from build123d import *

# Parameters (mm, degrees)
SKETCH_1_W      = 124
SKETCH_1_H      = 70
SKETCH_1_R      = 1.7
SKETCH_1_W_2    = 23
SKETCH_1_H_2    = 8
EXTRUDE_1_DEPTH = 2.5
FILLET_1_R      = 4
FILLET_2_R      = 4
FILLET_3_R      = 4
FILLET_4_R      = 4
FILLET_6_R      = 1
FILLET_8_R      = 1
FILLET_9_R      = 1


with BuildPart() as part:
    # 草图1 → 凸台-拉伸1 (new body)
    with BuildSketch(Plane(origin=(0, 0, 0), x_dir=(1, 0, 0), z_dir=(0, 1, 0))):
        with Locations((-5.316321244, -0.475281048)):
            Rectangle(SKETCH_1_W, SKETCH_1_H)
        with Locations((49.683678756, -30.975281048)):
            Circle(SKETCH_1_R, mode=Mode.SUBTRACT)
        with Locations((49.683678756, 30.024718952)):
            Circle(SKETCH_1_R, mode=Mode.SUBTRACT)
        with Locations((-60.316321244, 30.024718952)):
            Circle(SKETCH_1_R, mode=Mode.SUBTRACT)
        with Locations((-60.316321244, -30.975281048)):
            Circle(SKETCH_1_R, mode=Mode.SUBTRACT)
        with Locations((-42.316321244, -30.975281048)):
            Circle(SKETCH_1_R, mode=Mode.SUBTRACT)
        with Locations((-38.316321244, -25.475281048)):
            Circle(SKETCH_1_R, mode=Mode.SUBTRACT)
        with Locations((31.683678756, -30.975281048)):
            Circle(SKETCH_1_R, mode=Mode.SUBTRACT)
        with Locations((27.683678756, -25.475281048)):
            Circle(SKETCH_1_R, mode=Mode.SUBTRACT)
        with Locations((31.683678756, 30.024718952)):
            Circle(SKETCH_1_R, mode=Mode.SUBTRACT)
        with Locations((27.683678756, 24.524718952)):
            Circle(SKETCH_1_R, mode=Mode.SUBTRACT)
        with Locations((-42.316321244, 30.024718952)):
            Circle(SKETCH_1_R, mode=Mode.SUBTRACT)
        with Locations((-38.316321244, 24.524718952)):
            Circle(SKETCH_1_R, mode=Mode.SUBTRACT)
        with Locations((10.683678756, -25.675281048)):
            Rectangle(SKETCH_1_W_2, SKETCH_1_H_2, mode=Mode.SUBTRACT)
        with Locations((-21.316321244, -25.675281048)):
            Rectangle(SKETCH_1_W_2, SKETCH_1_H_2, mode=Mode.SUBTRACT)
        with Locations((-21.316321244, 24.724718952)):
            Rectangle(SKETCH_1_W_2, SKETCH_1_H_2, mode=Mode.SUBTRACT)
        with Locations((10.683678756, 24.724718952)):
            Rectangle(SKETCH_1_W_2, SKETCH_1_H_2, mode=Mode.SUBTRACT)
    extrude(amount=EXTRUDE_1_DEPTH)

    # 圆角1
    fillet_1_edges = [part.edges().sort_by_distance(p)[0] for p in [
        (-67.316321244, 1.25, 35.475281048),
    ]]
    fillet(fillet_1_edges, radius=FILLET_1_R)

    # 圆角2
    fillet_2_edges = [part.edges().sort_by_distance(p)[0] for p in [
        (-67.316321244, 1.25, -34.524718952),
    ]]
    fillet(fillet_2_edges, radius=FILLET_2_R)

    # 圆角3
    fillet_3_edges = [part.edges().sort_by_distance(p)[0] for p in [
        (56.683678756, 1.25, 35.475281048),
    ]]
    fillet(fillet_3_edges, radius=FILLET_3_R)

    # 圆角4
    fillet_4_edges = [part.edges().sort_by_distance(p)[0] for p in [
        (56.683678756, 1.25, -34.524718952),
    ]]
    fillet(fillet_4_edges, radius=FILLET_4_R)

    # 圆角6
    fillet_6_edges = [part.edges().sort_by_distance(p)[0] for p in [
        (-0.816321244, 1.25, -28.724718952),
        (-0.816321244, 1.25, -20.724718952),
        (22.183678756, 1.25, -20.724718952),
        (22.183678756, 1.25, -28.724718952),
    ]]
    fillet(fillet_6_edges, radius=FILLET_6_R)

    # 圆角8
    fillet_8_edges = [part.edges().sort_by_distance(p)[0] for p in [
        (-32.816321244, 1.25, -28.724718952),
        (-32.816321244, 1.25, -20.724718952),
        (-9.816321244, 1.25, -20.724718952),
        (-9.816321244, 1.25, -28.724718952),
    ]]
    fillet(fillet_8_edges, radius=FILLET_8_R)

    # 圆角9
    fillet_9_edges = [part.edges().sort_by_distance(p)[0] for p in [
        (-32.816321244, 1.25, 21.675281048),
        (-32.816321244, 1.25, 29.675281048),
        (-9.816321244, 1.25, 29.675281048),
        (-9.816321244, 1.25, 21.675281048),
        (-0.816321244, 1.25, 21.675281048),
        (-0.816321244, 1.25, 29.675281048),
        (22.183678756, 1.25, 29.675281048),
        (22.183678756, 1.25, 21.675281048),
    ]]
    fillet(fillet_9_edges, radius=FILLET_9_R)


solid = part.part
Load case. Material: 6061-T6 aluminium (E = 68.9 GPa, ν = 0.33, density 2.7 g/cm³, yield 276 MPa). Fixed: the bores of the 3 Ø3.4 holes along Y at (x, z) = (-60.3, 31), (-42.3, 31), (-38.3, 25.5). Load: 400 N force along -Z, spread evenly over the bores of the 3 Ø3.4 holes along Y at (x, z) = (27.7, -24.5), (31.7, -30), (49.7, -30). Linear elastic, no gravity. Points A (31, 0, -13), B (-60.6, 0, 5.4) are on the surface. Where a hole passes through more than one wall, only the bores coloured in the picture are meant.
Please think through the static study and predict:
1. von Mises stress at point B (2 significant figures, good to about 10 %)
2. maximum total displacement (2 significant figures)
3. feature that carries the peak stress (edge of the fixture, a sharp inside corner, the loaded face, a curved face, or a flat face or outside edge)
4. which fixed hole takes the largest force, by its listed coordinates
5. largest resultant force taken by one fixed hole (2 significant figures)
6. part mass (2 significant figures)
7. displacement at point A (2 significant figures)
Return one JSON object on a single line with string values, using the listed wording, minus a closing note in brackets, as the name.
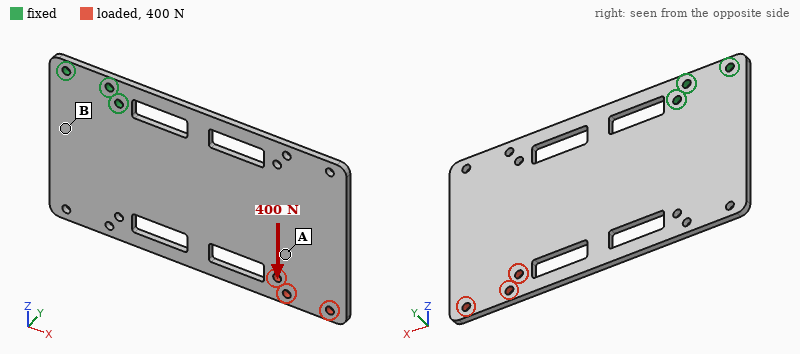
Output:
{"von Mises stress at point B": "20 MPa", "maximum total displacement": "0.18 mm", "feature that carries the peak stress": "a curved face", "which fixed hole takes the largest force, by its listed coordinates": "(-38.3, 25.5)", "largest resultant force taken by one fixed hole": "1.5 kN", "part mass": "53 g", "displacement at point A": "0.13 mm"}
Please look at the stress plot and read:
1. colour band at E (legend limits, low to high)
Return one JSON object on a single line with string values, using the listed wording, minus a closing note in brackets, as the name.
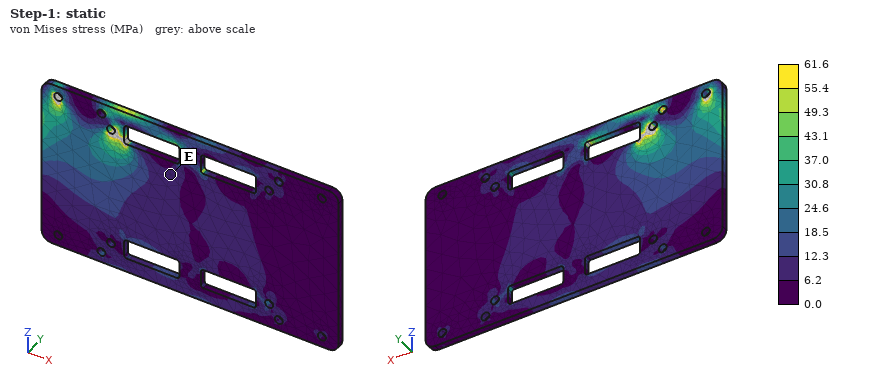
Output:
{"colour band at E": "6.2 to 12.3 MPa"}
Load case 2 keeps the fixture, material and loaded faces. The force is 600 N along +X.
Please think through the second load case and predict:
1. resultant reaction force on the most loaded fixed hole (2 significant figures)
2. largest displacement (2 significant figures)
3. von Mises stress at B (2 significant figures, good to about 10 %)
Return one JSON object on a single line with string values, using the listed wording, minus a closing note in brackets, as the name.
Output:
{"resultant reaction force on the most loaded fixed hole": "1.4 kN", "largest displacement": "0.17 mm", "von Mises stress at B": "20 MPa"}
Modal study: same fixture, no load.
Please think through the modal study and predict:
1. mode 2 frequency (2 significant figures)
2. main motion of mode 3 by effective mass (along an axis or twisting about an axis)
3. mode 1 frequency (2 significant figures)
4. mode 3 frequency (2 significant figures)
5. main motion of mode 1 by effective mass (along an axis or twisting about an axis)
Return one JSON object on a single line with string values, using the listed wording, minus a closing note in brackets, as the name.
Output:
{"mode 2 frequency": "400 Hz", "main motion of mode 3 by effective mass": "along Y", "mode 1 frequency": "160 Hz", "mode 3 frequency": "810 Hz", "main motion of mode 1 by effective mass": "along Y"}
